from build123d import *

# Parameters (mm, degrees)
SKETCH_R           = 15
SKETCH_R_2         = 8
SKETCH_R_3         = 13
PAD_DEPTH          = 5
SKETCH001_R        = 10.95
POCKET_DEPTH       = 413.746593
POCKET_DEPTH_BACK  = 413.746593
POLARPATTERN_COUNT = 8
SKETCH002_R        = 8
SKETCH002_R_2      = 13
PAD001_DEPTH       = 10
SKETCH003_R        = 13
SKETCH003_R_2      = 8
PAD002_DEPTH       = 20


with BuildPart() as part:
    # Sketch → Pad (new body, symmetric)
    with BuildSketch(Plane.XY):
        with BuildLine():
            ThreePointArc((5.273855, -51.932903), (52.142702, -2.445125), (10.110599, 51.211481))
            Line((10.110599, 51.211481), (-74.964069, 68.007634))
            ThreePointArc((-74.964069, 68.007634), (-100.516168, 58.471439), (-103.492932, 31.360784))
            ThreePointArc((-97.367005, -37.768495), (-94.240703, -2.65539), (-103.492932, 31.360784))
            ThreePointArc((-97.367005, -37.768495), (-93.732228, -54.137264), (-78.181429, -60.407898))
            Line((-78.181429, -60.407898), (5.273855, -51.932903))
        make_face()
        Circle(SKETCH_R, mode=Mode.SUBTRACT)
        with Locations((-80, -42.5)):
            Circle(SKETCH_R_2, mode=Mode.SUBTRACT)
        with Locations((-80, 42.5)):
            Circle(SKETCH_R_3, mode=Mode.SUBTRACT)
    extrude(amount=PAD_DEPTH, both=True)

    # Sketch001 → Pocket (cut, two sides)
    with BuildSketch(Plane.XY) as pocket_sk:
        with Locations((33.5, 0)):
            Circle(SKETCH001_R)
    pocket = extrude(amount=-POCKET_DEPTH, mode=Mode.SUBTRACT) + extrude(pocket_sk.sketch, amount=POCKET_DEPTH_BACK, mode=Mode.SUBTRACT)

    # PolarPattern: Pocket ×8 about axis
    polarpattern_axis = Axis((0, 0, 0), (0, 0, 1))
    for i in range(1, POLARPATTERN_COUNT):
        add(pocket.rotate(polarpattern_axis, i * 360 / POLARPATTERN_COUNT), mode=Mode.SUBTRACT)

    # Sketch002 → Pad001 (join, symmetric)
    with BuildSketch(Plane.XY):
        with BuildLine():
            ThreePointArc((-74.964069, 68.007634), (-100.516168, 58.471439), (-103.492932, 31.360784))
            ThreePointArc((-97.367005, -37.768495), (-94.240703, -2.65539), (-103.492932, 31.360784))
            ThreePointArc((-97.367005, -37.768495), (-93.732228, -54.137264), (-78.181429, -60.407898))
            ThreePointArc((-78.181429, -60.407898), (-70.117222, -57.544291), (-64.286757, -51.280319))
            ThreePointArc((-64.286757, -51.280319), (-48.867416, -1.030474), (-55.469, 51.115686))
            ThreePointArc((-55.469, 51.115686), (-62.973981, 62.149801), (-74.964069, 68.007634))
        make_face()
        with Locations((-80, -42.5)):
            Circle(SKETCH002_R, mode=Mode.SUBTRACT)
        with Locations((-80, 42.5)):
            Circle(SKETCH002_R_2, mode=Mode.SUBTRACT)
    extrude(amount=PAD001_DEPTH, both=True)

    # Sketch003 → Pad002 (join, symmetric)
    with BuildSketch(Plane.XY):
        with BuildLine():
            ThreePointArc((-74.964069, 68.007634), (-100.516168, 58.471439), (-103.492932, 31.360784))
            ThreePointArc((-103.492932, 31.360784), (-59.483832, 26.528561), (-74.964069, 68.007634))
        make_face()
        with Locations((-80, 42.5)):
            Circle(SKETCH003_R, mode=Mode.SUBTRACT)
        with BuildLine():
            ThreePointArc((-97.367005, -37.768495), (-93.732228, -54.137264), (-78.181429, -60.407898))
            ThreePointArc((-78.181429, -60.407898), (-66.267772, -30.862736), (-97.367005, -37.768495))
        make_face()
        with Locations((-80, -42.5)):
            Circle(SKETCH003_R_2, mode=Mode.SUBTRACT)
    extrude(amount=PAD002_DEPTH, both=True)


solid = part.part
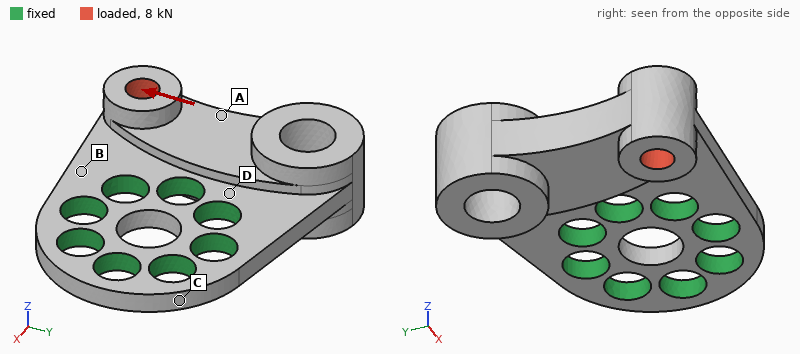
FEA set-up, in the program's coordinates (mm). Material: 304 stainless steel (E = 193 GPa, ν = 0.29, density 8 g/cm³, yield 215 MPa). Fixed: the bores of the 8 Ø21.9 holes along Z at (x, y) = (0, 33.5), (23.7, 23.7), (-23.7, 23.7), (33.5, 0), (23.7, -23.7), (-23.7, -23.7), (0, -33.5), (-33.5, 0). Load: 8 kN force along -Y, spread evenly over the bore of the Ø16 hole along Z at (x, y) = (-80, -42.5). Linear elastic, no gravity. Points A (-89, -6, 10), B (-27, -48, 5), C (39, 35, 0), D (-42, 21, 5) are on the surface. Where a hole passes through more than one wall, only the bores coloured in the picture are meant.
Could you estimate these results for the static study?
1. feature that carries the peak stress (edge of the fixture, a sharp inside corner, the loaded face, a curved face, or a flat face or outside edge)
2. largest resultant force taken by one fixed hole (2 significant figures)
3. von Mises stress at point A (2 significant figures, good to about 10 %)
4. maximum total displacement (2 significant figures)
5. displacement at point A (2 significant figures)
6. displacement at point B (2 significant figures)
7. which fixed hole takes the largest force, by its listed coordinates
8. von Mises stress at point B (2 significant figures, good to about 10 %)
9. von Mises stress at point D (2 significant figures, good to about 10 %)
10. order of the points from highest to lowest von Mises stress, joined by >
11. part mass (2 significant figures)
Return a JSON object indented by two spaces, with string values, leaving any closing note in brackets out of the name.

{
  "feature that carries the peak stress": "edge of the fixture",
  "largest resultant force taken by one fixed hole": "5.6 kN",
  "von Mises stress at point A": "8.6 MPa",
  "maximum total displacement": "9.7 µm",
  "displacement at point A": "6.1 µm",
  "displacement at point B": "1.5 µm",
  "which fixed hole takes the largest force, by its listed coordinates": "(-33.5, 0)",
  "von Mises stress at point B": "13 MPa",
  "von Mises stress at point D": "18 MPa",
  "order of the points from highest to lowest von Mises stress, joined by >": "D > B > A > C",
  "part mass": "1.7 kg"
}
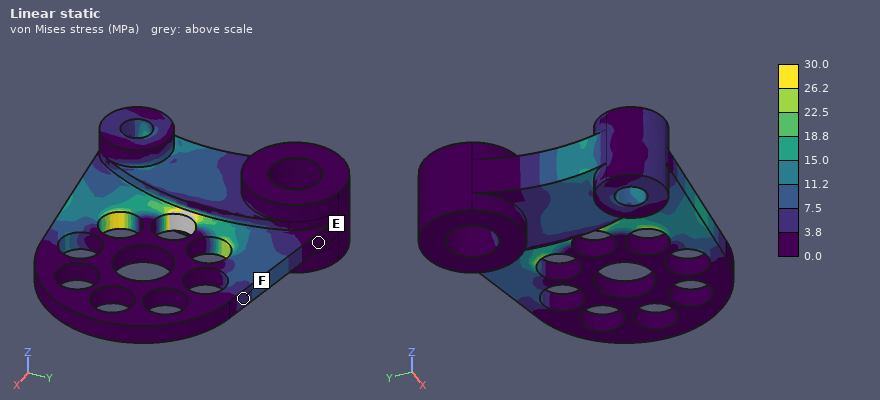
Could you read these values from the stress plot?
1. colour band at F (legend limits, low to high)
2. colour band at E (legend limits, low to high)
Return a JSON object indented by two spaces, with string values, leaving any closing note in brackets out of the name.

{
  "colour band at F": "3.8 to 7.5 MPa",
  "colour band at E": "0.0 to 3.8 MPa"
}
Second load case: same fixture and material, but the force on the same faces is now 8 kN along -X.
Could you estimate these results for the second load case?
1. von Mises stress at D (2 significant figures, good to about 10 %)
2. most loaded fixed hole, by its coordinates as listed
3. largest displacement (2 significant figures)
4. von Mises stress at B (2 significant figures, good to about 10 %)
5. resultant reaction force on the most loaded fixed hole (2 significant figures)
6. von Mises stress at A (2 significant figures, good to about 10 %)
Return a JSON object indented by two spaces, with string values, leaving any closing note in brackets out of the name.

{
  "von Mises stress at D": "5.4 MPa",
  "most loaded fixed hole, by its coordinates as listed": "(-23.7, -23.7)",
  "largest displacement": "8.3 µm",
  "von Mises stress at B": "15 MPa",
  "resultant reaction force on the most loaded fixed hole": "5.6 kN",
  "von Mises stress at A": "5.5 MPa"
}
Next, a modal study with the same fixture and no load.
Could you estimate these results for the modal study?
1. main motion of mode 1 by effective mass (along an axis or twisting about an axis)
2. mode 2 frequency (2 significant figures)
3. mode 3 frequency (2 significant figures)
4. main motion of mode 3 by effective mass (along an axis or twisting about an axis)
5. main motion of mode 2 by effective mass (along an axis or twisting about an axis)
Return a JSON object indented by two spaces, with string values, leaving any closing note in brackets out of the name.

{
  "main motion of mode 1 by effective mass": "along Z",
  "mode 2 frequency": "2300 Hz",
  "mode 3 frequency": "5200 Hz",
  "main motion of mode 3 by effective mass": "along Y",
  "main motion of mode 2 by effective mass": "twisting about X"
}
